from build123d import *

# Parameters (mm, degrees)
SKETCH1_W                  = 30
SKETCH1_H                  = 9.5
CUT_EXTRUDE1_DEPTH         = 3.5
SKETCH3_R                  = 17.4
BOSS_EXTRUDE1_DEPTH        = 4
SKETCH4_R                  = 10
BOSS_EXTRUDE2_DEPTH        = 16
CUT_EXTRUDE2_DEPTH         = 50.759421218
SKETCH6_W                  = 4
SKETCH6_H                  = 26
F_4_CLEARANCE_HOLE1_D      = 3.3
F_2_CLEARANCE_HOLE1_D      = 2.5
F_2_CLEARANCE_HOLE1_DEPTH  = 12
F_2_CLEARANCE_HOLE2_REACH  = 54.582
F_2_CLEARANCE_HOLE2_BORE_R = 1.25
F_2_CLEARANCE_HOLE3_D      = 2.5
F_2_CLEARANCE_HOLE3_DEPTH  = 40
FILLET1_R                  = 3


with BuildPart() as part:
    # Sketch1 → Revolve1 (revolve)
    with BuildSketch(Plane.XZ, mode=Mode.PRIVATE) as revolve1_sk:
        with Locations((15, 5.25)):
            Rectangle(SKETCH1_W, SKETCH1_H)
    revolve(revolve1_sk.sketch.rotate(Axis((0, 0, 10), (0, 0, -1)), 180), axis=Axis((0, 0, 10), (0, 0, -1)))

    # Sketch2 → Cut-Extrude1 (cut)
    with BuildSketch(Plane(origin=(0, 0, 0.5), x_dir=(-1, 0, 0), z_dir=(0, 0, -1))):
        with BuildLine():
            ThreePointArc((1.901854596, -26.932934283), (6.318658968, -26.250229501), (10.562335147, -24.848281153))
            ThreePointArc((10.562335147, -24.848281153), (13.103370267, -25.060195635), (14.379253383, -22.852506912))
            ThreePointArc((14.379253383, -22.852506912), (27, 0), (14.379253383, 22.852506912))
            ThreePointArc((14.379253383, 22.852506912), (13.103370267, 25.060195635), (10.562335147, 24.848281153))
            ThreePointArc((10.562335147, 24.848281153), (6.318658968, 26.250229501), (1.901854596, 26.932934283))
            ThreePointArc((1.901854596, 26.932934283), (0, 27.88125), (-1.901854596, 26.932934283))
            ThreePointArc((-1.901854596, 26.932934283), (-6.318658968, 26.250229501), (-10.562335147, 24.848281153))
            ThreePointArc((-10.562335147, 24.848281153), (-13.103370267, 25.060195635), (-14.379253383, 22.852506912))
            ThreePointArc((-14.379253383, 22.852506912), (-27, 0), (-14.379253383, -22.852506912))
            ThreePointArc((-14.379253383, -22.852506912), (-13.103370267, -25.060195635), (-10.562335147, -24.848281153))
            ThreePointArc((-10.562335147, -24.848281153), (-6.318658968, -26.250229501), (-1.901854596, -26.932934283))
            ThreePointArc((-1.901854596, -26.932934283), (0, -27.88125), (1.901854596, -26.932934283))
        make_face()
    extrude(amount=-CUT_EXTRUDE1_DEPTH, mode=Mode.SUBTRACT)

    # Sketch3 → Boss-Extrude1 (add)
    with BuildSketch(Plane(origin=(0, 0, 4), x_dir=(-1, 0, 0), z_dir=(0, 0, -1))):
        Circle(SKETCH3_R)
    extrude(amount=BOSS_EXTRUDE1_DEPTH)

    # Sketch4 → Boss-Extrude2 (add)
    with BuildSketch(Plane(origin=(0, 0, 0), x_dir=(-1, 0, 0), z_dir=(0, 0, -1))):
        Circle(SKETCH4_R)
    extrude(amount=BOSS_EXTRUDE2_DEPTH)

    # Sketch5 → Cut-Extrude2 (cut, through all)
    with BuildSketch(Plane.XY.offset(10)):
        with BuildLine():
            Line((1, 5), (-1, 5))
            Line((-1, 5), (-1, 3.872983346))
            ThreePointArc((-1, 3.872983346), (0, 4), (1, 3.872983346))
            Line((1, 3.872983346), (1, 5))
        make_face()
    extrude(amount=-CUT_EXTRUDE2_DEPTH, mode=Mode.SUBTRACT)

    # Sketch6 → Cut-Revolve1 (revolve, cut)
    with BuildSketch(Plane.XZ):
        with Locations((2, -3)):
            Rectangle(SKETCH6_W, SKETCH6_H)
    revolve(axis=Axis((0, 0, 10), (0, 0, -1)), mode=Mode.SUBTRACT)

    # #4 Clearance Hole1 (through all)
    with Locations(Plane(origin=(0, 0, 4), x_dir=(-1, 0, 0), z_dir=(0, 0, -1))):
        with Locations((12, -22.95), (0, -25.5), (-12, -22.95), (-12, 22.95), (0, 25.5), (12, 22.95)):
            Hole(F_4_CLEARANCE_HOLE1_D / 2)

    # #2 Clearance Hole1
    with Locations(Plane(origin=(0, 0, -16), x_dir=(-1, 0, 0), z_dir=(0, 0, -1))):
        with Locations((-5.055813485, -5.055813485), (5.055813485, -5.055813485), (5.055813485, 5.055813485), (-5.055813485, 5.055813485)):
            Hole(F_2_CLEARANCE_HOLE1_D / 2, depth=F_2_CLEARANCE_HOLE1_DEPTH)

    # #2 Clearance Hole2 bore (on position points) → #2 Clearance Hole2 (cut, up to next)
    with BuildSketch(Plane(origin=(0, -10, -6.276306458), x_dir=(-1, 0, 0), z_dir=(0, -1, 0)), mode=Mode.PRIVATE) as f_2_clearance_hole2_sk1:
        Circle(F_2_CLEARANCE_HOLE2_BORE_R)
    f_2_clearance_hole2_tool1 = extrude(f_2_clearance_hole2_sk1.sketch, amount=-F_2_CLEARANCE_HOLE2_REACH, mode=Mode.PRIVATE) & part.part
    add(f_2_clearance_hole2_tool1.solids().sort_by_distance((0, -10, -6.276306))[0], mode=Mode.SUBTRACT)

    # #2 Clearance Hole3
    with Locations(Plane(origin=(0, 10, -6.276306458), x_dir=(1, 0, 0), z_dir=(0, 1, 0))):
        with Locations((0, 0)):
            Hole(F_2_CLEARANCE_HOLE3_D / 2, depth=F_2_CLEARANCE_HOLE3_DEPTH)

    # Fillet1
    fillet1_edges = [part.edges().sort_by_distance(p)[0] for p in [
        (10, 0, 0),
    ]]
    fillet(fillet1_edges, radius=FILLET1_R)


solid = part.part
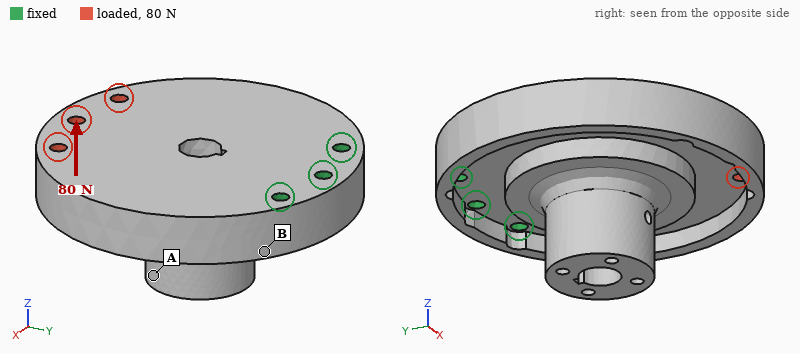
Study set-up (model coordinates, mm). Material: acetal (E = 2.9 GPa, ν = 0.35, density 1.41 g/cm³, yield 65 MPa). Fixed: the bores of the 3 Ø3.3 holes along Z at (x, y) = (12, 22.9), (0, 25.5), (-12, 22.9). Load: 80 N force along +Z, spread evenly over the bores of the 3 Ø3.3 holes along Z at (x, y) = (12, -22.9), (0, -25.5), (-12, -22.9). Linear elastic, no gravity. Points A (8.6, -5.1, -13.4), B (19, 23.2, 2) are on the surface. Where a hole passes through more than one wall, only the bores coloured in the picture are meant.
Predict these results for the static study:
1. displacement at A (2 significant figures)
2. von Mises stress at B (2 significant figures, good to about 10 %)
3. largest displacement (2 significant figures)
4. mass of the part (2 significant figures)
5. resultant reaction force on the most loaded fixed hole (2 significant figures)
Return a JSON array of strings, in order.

["0.52 mm", "4.7 MPa", "0.88 mm", "36 g", "63 N"]
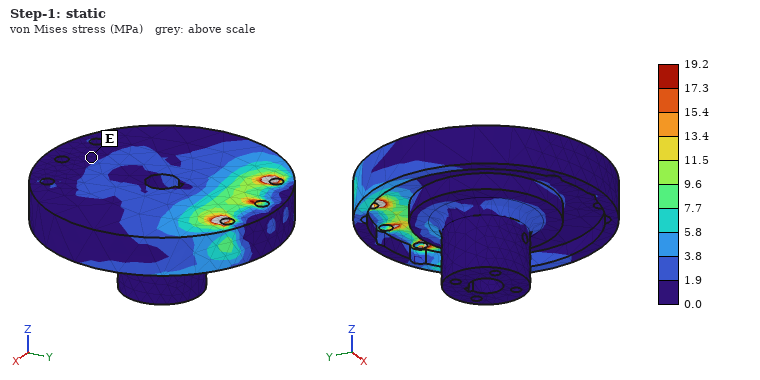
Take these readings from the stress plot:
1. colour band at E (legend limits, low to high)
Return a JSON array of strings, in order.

["0.0 to 1.9 MPa"]
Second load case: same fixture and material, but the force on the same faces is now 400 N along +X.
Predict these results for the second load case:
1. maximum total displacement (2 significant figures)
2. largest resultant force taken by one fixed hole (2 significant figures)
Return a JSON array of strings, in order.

["0.29 mm", "730 N"]
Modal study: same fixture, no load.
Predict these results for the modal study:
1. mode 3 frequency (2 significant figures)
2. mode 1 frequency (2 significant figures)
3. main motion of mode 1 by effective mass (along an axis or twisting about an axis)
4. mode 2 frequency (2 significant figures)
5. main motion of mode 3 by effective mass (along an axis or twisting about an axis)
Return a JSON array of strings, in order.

["1800 Hz", "500 Hz", "along Z", "1500 Hz", "along X"]
